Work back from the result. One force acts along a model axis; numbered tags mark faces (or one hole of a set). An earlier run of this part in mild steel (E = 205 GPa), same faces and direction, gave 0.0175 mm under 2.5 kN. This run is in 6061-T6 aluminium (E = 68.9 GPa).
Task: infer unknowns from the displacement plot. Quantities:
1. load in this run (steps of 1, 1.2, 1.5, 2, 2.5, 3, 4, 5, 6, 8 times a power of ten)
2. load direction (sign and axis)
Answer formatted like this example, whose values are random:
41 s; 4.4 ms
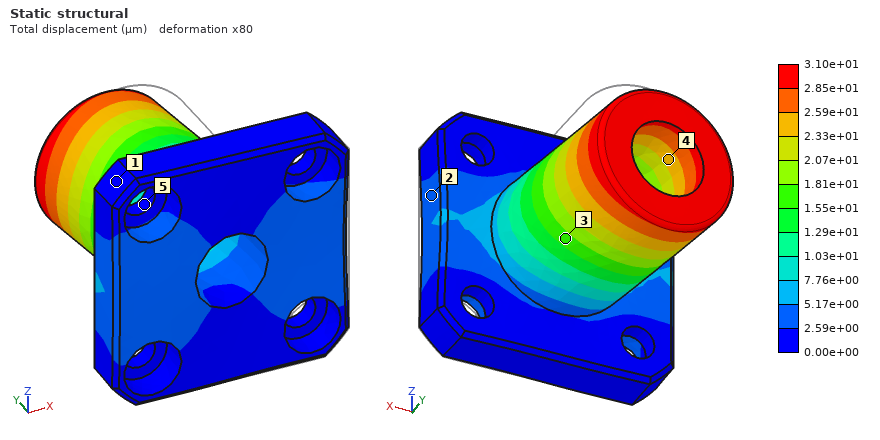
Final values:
1.5 kN; -X
